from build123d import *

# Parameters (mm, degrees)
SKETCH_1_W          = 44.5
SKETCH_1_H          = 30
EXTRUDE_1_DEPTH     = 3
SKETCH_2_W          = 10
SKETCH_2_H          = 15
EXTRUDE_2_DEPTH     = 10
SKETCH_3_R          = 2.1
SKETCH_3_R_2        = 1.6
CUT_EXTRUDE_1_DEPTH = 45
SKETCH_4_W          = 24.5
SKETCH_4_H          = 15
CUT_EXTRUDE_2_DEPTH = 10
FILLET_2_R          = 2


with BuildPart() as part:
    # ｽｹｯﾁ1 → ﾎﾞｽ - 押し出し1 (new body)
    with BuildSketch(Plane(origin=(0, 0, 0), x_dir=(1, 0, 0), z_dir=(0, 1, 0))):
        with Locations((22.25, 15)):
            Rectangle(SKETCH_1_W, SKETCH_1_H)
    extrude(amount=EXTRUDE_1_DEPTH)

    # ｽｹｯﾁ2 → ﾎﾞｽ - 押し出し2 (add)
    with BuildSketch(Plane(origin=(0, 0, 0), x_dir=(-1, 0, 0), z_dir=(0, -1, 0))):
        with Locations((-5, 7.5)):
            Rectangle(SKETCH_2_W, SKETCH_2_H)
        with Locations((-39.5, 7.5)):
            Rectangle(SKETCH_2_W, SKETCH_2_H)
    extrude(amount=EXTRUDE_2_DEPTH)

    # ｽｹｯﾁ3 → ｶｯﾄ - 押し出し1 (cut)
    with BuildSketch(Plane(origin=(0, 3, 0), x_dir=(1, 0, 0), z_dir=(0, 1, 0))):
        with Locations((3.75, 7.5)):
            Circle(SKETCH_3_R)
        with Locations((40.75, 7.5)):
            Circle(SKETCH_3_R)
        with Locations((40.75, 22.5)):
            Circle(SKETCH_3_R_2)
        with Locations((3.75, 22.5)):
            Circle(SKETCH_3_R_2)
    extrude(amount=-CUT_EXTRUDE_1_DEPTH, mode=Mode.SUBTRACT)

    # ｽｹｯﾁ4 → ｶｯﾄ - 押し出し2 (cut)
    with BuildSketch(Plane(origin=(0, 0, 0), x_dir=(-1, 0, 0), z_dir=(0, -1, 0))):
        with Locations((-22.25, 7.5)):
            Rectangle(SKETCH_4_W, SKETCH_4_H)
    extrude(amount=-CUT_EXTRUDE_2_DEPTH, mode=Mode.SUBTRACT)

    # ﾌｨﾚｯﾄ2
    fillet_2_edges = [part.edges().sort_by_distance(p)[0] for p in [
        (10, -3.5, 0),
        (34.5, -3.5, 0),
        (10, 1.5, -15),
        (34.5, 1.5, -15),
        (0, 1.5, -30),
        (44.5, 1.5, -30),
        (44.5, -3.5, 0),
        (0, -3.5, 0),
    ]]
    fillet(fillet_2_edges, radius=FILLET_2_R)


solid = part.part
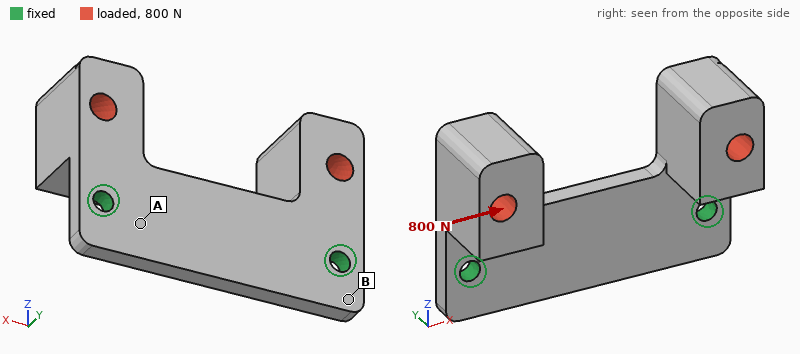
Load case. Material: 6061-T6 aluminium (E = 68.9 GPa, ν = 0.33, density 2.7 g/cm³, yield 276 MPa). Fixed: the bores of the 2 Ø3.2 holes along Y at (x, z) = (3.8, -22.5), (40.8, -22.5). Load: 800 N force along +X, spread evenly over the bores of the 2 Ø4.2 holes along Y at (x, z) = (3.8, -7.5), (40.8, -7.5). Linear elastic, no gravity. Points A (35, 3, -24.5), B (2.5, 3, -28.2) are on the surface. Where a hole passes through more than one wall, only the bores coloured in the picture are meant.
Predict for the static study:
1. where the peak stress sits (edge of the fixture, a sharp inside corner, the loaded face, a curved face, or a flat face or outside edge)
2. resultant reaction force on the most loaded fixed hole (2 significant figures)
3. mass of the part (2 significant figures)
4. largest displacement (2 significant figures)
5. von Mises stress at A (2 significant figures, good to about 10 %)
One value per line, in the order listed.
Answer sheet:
a curved face
490 N
15 g
71 µm
29 MPa
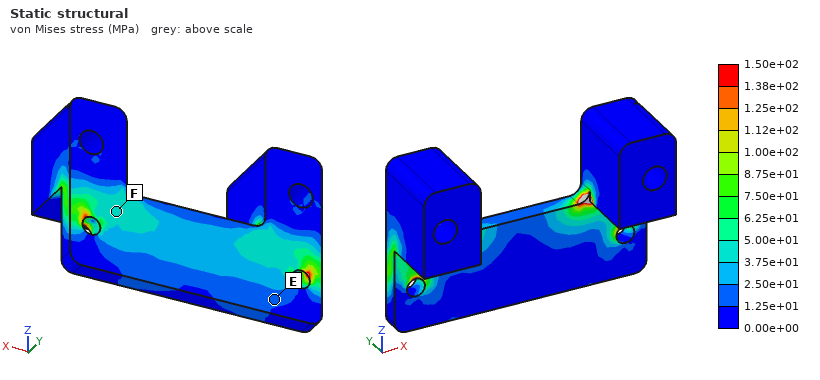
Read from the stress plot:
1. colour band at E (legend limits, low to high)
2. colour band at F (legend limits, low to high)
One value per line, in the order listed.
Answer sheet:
1.25e+01 to 2.50e+01 MPa
3.75e+01 to 5.00e+01 MPa
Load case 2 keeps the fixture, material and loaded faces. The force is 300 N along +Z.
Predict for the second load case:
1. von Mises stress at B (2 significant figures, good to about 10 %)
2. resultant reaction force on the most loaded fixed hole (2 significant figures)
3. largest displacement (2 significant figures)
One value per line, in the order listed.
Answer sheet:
5.3 MPa
150 N
73 µm
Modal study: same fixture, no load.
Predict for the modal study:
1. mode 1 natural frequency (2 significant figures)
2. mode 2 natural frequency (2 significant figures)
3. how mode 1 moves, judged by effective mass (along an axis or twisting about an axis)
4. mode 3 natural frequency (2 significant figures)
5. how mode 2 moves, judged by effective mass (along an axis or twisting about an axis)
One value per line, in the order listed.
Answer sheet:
2600 Hz
2700 Hz
along Y
5700 Hz
twisting about Z
